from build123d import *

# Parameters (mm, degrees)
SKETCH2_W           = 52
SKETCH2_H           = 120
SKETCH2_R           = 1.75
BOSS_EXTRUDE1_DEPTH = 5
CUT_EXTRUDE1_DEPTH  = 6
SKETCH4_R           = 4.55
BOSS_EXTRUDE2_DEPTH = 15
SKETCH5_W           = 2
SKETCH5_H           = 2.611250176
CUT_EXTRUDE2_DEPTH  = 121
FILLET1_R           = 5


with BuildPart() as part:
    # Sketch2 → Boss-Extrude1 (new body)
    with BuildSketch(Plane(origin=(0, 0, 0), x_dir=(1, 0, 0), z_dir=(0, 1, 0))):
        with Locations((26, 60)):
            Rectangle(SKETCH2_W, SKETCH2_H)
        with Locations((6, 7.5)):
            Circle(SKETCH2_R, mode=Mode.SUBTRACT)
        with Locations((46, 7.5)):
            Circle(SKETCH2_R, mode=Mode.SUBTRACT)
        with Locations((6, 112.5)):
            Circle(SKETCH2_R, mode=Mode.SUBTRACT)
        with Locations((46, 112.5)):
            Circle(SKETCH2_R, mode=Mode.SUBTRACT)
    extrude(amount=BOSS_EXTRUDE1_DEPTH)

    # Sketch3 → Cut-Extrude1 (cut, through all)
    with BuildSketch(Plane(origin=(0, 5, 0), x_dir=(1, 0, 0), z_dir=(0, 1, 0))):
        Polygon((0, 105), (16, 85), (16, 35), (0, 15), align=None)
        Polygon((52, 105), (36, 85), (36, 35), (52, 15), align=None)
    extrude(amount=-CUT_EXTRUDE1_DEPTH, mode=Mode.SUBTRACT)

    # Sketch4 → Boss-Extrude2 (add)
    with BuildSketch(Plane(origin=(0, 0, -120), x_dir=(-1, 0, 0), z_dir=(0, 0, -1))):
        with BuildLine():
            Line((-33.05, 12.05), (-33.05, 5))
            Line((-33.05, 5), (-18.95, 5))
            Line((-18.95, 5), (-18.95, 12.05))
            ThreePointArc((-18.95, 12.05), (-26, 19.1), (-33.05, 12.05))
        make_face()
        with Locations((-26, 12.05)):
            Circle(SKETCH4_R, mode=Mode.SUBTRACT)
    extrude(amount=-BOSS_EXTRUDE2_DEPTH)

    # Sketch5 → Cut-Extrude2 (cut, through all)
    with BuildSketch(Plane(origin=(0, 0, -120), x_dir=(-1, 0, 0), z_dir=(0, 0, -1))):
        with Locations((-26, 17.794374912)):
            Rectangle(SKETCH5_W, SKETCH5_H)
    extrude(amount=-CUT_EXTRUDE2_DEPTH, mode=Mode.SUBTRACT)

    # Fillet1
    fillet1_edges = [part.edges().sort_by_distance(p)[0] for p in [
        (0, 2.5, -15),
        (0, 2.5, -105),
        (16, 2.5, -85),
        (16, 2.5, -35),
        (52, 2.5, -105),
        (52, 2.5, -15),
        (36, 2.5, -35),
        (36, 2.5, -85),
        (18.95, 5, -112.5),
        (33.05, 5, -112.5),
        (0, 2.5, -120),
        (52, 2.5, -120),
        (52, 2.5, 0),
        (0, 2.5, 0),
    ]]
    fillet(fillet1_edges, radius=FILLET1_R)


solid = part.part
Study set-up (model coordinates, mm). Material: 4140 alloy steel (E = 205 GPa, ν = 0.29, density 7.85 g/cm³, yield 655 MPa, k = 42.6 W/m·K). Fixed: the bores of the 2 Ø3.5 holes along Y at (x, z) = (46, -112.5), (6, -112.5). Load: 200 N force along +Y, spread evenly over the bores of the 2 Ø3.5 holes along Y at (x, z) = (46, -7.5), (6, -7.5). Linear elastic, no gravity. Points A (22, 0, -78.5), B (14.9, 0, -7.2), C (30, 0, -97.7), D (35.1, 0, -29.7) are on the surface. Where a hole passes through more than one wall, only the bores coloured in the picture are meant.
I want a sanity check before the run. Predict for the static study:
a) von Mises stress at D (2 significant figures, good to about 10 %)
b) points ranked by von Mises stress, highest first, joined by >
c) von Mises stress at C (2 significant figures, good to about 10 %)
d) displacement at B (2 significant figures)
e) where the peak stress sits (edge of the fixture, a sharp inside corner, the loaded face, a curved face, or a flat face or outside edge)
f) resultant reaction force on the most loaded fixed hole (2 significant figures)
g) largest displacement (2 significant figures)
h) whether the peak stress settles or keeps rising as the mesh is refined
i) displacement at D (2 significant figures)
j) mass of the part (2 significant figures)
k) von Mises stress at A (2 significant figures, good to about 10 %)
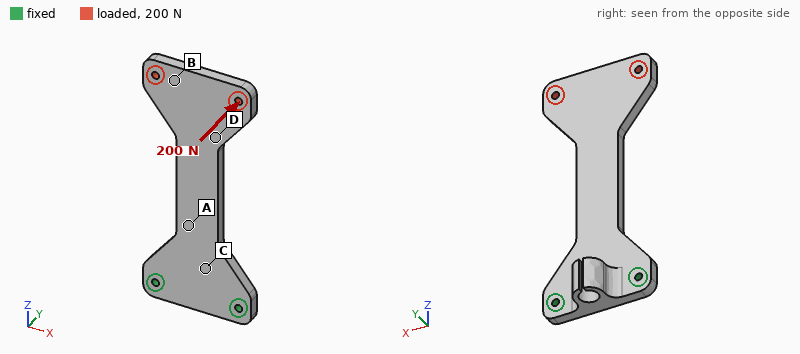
40 MPa
A > C > D > B
120 MPa
1.4 mm
edge of the fixture
110 N
1.6 mm
keeps rising
0.94 mm
170 g
170 MPa
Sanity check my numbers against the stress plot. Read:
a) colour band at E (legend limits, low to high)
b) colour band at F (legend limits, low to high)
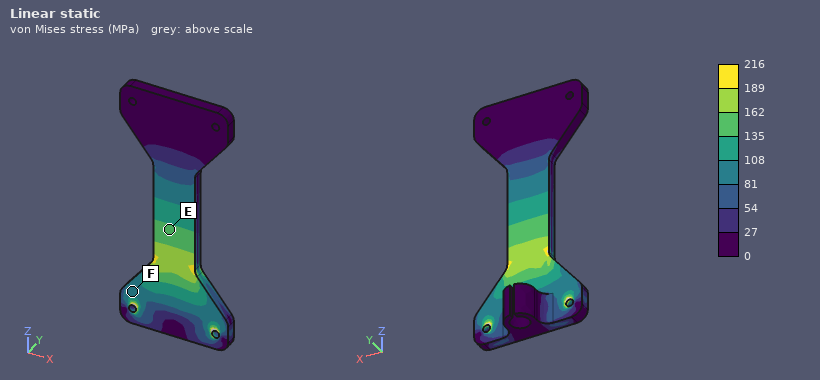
135 to 162 MPa
81 to 108 MPa
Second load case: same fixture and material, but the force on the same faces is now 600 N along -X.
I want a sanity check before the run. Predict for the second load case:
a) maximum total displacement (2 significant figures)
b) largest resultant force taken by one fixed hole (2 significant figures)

0.23 mm
1.6 kN
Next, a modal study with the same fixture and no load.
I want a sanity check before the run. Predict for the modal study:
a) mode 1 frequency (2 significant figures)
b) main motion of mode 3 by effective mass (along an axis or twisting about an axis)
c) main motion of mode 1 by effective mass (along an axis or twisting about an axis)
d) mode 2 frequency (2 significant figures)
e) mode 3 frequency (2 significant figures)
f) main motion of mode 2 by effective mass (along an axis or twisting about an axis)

270 Hz
twisting about Z
along Y
1200 Hz
1400 Hz
along X
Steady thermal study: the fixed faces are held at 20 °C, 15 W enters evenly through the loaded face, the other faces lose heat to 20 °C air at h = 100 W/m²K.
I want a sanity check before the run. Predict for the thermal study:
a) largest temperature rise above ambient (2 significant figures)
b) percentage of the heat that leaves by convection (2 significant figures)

52 K
97 %
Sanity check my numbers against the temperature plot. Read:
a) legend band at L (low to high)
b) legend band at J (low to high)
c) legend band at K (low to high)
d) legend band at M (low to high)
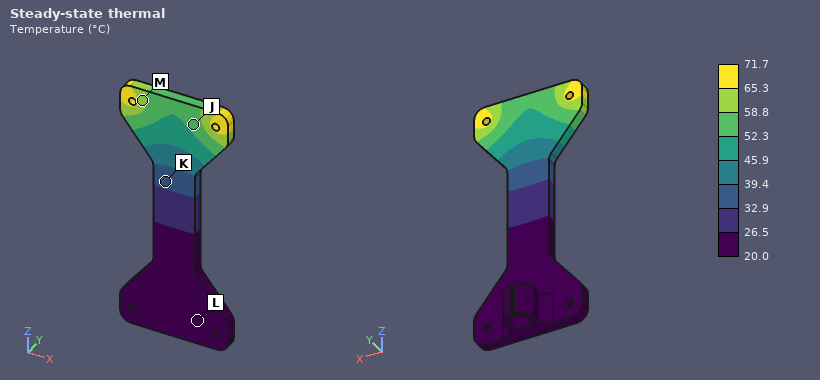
20.0 to 26.5 °C
52.3 to 58.8 °C
32.9 to 39.4 °C
58.8 to 65.3 °C
